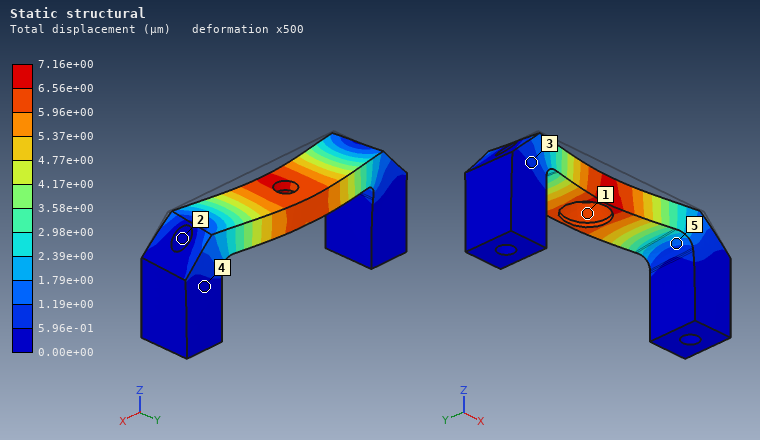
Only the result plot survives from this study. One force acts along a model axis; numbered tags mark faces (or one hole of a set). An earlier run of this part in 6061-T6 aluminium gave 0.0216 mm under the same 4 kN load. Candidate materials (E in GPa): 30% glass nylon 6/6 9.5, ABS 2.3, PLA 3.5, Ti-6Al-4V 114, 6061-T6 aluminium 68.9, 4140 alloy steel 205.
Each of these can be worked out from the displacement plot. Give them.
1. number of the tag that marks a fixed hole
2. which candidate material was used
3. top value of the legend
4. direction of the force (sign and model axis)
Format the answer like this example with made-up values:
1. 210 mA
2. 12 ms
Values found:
1. 2
2. 4140 alloy steel
3. 7.16e+00 µm
4. +Y
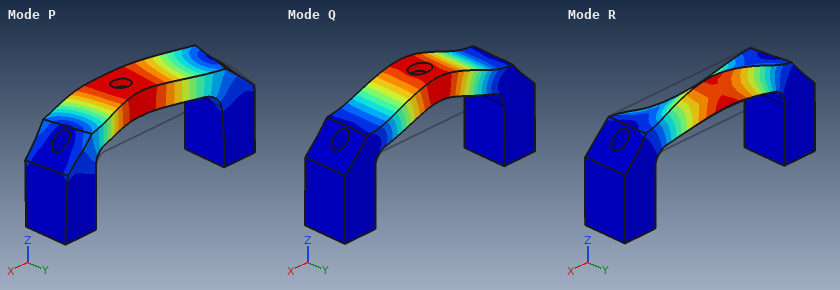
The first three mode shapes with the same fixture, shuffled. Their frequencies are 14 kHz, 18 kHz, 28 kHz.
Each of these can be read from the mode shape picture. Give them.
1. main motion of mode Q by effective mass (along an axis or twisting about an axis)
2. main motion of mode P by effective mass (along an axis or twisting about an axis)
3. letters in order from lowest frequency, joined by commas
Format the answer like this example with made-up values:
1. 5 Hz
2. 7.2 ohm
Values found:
1. along Z
2. along Y
3. Q, P, R
